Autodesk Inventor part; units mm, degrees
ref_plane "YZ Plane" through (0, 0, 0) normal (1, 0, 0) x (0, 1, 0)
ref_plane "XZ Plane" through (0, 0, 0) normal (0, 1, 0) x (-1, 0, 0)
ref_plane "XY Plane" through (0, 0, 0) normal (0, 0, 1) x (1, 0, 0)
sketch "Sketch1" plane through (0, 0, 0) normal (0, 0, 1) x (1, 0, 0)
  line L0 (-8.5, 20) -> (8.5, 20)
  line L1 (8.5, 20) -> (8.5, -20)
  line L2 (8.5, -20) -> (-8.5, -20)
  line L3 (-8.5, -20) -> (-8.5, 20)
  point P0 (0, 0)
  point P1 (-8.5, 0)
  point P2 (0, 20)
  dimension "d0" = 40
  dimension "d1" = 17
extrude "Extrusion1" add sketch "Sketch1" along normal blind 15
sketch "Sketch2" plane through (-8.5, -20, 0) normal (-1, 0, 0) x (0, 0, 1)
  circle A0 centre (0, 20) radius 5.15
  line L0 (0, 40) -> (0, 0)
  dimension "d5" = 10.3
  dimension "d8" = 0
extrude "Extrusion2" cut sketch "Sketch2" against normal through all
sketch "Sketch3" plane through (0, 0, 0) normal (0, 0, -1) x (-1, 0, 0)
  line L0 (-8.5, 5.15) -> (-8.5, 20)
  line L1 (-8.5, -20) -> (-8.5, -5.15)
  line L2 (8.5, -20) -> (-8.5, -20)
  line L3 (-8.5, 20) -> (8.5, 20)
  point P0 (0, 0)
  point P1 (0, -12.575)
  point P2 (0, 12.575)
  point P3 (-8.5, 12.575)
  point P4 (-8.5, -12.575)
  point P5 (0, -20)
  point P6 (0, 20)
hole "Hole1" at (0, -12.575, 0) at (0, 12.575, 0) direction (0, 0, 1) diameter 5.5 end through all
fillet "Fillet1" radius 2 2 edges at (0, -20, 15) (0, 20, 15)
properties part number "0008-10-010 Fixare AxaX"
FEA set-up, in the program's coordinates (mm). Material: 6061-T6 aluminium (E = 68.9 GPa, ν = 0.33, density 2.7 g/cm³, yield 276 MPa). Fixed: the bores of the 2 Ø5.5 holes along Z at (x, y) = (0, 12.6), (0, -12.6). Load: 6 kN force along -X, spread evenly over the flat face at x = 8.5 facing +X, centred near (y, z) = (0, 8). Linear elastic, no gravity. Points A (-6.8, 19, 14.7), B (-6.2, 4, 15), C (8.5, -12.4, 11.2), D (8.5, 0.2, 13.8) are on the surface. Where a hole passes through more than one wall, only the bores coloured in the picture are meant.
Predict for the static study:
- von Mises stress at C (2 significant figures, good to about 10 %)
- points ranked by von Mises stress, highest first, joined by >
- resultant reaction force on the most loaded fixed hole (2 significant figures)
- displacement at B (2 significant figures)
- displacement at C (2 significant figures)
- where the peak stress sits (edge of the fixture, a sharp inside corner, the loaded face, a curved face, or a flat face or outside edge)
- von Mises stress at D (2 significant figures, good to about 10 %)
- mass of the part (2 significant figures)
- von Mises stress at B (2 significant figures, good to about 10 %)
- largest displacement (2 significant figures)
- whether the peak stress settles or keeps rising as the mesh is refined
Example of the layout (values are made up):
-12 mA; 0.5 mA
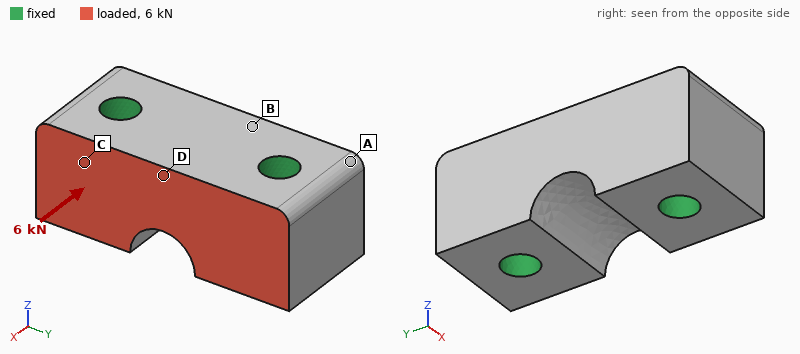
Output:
17 MPa; C > D > B > A; 3.0 kN; 1.7 µm; 1.2 µm; edge of the fixture; 11 MPa; 24 g; 5.8 MPa; 3.4 µm; keeps rising
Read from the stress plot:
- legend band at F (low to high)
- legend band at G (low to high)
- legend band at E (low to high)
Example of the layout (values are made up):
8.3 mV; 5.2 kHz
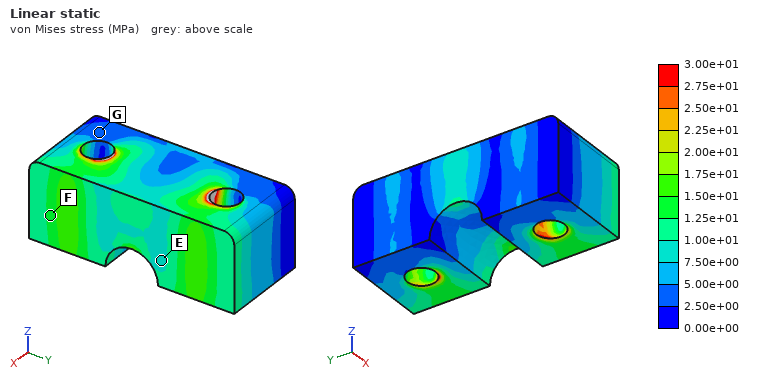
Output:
1.25e+01 to 1.50e+01 MPa; 2.50e+00 to 5.00e+00 MPa; 7.50e+00 to 1.00e+01 MPa
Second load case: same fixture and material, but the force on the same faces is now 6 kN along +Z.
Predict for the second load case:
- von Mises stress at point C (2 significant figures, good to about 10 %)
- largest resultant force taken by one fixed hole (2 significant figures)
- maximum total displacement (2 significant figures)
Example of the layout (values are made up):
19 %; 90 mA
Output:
24 MPa; 3.0 kN; 10 µm
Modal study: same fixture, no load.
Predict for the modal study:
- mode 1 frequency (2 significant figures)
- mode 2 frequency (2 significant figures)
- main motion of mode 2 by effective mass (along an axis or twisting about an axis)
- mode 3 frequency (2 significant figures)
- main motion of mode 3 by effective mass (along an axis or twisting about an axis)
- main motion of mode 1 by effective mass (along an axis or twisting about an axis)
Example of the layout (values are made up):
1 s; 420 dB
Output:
52 kHz; 57 kHz; along Z; 65 kHz; twisting about Y; along X
